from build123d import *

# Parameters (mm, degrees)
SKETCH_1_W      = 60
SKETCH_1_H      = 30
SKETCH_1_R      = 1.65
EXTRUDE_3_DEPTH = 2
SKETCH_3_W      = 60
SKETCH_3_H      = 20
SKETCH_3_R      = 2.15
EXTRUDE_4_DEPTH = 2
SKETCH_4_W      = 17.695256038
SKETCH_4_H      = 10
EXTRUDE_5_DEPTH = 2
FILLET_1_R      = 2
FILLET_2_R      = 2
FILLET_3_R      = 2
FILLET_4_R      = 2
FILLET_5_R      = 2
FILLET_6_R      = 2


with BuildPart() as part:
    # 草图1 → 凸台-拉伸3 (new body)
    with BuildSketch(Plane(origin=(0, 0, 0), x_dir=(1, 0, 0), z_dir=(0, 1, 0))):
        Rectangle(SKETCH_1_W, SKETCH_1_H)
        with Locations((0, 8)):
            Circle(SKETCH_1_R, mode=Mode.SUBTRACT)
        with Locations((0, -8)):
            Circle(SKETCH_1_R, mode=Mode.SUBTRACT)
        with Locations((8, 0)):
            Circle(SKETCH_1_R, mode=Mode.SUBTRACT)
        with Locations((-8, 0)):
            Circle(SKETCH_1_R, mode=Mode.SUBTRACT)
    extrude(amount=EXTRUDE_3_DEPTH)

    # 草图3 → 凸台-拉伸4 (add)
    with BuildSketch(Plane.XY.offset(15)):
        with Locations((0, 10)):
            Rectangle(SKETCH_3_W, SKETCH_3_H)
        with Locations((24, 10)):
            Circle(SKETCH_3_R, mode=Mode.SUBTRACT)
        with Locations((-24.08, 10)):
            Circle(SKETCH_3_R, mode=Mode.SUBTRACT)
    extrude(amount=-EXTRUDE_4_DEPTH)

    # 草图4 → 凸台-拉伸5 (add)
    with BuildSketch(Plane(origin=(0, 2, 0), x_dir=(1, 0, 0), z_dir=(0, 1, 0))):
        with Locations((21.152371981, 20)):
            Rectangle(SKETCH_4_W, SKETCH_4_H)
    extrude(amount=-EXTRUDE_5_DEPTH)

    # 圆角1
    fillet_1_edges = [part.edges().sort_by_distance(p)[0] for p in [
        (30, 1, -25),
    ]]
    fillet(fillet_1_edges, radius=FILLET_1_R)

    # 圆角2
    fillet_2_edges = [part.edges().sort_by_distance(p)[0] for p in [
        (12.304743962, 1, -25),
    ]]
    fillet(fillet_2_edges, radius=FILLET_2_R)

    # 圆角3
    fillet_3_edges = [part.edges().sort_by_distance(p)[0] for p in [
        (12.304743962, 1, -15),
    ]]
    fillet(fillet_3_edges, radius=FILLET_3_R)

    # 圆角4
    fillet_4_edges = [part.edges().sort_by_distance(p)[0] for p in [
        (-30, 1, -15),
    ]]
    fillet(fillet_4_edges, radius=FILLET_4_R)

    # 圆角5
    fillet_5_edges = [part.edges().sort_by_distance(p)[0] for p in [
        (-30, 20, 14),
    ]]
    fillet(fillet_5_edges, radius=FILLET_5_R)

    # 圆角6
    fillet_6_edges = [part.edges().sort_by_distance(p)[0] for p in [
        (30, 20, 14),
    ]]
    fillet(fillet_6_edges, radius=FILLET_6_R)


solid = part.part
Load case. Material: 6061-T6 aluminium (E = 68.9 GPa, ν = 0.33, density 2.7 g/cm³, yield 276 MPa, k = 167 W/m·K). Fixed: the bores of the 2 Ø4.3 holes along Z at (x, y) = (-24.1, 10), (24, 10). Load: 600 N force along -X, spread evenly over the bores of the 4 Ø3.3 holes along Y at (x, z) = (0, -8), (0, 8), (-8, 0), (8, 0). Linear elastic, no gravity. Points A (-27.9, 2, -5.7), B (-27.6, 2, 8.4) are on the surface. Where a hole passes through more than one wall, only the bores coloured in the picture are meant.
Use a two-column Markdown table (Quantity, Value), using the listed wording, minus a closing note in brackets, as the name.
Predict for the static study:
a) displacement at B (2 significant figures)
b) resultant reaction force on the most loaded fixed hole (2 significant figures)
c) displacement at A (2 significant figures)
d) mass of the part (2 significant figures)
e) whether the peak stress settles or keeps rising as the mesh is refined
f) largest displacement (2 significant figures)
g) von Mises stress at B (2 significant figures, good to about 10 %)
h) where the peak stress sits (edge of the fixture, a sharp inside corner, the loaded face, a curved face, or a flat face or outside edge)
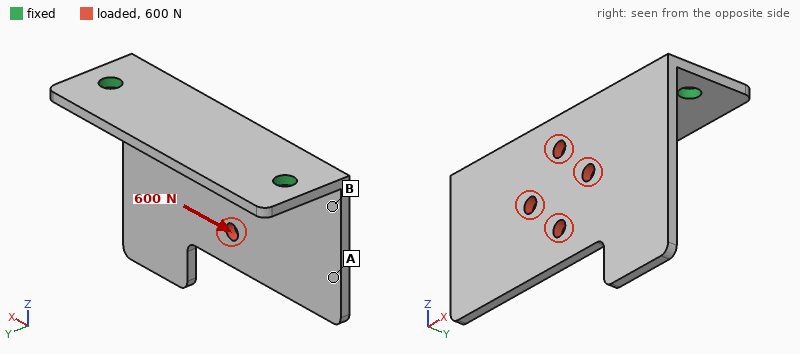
| Quantity | Value |
|---|---|
| displacement at B | 0.041 mm |
| resultant reaction force on the most loaded fixed hole | 360 N |
| displacement at A | 0.077 mm |
| mass of the part | 16 g |
| whether the peak stress settles or keeps rising as the mesh is refined | keeps rising |
| largest displacement | 0.11 mm |
| von Mises stress at B | 26 MPa |
| where the peak stress sits | edge of the fixture |
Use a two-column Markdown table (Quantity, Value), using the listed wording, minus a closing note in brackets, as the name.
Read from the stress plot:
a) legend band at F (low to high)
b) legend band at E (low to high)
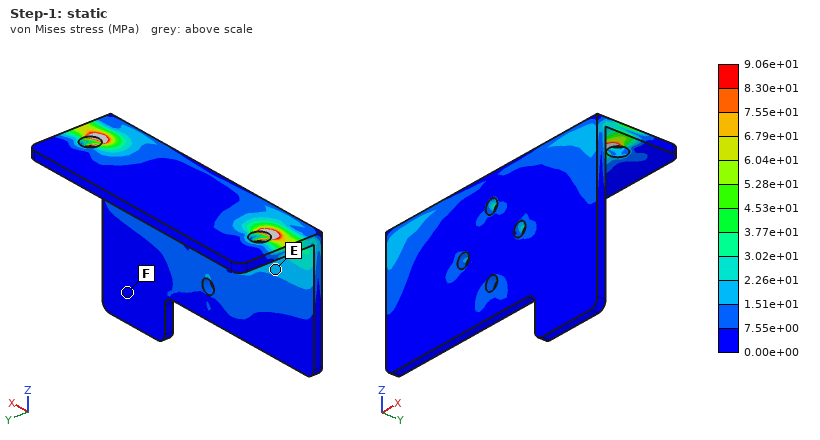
| Quantity | Value |
|---|---|
| legend band at F | 0.00e+00 to 7.55e+00 MPa |
| legend band at E | 1.51e+01 to 2.26e+01 MPa |
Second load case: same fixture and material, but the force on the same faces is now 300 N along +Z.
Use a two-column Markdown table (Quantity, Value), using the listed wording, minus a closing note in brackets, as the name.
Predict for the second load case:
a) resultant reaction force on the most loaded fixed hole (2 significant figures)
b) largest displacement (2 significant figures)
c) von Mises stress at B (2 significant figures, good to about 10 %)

| Quantity | Value |
|---|---|
| resultant reaction force on the most loaded fixed hole | 160 N |
| largest displacement | 0.20 mm |
| von Mises stress at B | 11 MPa |
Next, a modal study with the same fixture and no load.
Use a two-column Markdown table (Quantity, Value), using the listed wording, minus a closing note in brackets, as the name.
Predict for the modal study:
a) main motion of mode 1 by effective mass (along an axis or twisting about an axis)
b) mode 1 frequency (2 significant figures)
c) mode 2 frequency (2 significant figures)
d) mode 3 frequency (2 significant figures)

| Quantity | Value |
|---|---|
| main motion of mode 1 by effective mass | along Y |
| mode 1 frequency | 1000 Hz |
| mode 2 frequency | 2000 Hz |
| mode 3 frequency | 4500 Hz |
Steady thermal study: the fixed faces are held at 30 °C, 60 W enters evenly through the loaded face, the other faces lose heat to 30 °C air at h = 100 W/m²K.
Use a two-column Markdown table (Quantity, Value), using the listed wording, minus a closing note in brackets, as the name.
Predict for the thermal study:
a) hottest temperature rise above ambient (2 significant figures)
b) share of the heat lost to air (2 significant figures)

| Quantity | Value |
|---|---|
| hottest temperature rise above ambient | 79 K |
| share of the heat lost to air | 40 % |
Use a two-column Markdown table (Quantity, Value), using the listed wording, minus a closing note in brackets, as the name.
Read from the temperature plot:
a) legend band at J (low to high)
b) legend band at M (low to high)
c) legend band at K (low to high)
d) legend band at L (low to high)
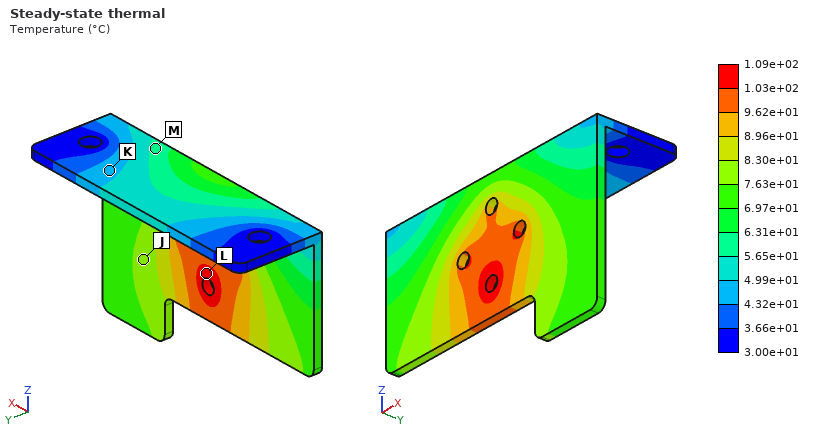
| Quantity | Value |
|---|---|
| legend band at J | 7.63e+01 to 8.30e+01 °C |
| legend band at M | 5.65e+01 to 6.31e+01 °C |
| legend band at K | 4.32e+01 to 4.99e+01 °C |
| legend band at L | 1.03e+02 to 1.09e+02 °C |
